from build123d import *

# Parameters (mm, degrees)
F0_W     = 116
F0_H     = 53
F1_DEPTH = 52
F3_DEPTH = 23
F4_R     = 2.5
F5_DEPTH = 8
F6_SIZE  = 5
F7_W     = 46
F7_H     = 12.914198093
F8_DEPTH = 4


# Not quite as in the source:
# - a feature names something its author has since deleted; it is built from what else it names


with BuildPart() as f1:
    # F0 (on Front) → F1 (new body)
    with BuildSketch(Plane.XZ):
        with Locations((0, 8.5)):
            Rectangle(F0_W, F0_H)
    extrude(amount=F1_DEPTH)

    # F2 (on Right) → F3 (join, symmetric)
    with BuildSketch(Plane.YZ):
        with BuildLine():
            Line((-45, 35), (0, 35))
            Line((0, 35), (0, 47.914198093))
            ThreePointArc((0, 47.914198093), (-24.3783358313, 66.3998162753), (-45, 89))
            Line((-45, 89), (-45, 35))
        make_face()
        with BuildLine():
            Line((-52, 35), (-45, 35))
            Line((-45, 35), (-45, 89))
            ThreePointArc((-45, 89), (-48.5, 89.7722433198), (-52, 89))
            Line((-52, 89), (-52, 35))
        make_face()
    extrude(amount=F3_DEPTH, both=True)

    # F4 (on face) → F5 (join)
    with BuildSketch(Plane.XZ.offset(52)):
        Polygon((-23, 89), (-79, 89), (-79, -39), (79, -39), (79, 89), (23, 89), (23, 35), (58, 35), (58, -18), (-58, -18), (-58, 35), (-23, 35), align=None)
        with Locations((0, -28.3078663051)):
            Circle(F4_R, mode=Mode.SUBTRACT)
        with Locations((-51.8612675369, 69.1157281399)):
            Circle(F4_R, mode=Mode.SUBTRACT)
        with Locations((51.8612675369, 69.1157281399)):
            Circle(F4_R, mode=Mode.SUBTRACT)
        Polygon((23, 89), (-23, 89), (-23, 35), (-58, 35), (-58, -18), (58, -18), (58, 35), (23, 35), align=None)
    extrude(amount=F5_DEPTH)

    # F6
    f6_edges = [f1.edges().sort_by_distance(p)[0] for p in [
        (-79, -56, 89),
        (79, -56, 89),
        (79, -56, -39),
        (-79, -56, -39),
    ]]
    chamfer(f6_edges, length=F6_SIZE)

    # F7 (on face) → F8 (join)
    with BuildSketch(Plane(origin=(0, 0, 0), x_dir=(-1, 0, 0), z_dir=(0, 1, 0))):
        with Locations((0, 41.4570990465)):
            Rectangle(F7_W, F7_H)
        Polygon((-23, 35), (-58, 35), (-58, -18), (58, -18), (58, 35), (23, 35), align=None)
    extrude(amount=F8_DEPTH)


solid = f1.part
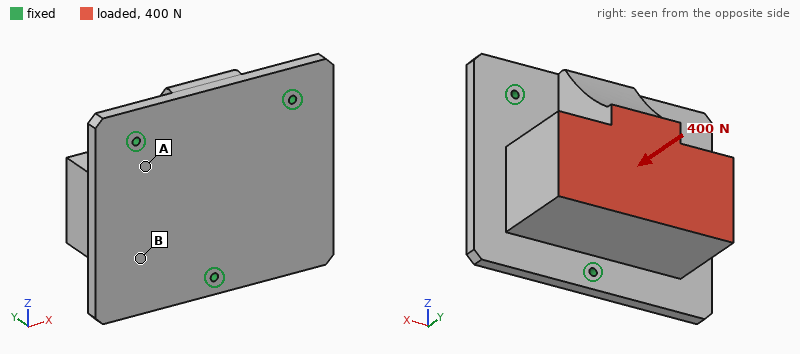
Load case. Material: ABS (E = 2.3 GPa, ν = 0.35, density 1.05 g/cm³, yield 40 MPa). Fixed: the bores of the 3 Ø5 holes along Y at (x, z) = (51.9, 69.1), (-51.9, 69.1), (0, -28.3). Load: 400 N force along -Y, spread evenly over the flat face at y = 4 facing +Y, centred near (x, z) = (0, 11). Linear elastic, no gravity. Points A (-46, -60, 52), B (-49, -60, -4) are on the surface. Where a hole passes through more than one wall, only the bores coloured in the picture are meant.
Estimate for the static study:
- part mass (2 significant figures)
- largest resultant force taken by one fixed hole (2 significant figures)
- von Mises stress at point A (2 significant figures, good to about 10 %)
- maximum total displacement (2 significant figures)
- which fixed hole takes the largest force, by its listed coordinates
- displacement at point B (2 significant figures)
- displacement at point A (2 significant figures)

620 g
250 N
0.57 MPa
55 µm
(0, -28.3)
50 µm
31 µm
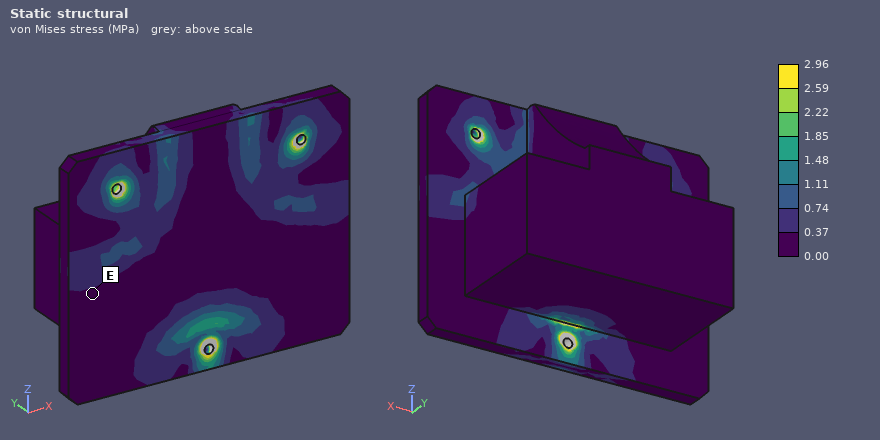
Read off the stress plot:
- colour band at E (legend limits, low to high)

0.00 to 0.37 MPa
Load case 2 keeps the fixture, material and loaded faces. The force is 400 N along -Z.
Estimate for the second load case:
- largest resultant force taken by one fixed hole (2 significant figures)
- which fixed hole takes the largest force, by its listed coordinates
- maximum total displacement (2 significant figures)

330 N
(0, -28.3)
0.13 mm
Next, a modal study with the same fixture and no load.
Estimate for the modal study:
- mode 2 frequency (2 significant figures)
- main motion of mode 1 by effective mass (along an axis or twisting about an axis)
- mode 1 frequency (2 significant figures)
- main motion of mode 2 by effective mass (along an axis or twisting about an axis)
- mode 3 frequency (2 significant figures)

550 Hz
along X
370 Hz
along Y
690 Hz
